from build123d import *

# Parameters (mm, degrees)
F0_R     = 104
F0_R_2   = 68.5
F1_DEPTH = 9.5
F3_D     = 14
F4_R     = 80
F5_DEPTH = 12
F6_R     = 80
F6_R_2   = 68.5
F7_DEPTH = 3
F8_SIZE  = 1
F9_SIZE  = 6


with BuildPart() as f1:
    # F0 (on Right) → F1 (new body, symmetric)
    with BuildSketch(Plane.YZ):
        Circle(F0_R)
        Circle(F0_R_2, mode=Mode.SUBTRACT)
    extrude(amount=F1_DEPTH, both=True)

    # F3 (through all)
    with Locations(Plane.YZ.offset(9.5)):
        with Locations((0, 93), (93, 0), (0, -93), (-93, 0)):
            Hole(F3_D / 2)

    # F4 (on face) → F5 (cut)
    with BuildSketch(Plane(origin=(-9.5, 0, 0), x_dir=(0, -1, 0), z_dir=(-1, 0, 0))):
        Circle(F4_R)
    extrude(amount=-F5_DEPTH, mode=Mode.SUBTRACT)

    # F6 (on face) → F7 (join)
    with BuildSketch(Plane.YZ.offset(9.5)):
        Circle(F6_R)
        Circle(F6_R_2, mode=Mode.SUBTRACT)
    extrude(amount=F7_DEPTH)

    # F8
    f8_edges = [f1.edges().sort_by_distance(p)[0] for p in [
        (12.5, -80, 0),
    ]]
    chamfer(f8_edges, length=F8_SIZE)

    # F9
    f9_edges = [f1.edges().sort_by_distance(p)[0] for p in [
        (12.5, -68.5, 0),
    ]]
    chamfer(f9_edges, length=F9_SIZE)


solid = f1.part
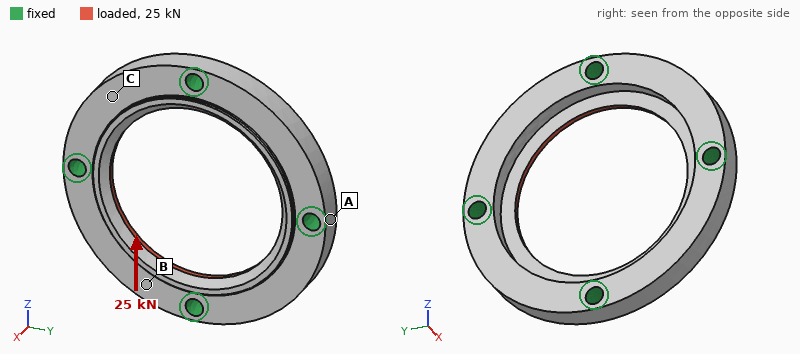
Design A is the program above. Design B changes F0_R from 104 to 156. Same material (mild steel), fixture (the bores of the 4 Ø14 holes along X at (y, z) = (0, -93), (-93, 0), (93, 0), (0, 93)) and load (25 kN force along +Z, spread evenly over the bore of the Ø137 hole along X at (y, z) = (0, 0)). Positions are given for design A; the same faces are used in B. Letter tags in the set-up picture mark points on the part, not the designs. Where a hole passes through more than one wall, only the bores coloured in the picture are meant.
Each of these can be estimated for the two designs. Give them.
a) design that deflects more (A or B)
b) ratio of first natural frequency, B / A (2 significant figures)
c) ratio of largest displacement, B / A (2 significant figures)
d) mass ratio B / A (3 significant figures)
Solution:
A
0.36
0.63
3.71
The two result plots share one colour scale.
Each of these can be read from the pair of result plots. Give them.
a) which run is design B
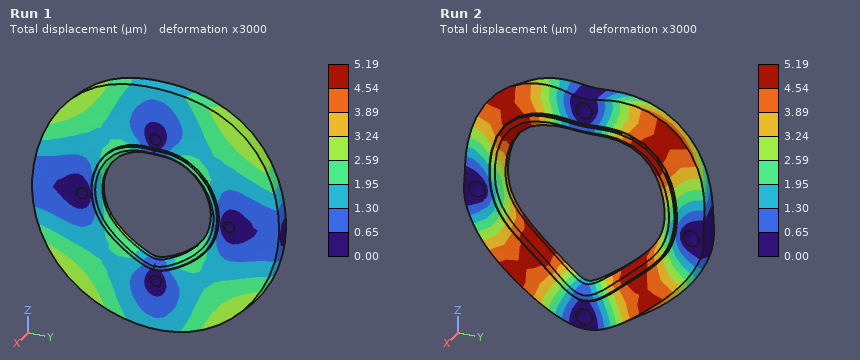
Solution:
Run 1
